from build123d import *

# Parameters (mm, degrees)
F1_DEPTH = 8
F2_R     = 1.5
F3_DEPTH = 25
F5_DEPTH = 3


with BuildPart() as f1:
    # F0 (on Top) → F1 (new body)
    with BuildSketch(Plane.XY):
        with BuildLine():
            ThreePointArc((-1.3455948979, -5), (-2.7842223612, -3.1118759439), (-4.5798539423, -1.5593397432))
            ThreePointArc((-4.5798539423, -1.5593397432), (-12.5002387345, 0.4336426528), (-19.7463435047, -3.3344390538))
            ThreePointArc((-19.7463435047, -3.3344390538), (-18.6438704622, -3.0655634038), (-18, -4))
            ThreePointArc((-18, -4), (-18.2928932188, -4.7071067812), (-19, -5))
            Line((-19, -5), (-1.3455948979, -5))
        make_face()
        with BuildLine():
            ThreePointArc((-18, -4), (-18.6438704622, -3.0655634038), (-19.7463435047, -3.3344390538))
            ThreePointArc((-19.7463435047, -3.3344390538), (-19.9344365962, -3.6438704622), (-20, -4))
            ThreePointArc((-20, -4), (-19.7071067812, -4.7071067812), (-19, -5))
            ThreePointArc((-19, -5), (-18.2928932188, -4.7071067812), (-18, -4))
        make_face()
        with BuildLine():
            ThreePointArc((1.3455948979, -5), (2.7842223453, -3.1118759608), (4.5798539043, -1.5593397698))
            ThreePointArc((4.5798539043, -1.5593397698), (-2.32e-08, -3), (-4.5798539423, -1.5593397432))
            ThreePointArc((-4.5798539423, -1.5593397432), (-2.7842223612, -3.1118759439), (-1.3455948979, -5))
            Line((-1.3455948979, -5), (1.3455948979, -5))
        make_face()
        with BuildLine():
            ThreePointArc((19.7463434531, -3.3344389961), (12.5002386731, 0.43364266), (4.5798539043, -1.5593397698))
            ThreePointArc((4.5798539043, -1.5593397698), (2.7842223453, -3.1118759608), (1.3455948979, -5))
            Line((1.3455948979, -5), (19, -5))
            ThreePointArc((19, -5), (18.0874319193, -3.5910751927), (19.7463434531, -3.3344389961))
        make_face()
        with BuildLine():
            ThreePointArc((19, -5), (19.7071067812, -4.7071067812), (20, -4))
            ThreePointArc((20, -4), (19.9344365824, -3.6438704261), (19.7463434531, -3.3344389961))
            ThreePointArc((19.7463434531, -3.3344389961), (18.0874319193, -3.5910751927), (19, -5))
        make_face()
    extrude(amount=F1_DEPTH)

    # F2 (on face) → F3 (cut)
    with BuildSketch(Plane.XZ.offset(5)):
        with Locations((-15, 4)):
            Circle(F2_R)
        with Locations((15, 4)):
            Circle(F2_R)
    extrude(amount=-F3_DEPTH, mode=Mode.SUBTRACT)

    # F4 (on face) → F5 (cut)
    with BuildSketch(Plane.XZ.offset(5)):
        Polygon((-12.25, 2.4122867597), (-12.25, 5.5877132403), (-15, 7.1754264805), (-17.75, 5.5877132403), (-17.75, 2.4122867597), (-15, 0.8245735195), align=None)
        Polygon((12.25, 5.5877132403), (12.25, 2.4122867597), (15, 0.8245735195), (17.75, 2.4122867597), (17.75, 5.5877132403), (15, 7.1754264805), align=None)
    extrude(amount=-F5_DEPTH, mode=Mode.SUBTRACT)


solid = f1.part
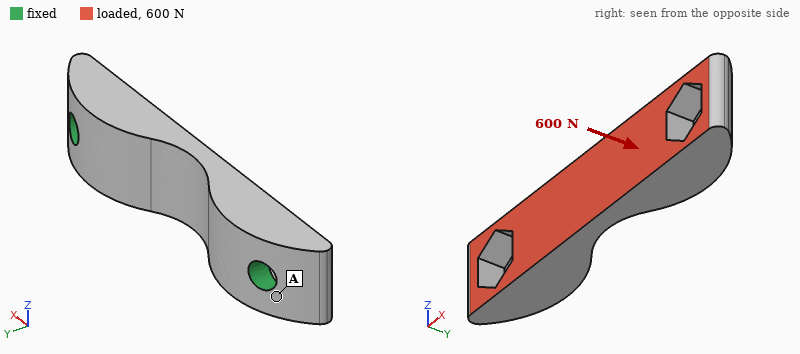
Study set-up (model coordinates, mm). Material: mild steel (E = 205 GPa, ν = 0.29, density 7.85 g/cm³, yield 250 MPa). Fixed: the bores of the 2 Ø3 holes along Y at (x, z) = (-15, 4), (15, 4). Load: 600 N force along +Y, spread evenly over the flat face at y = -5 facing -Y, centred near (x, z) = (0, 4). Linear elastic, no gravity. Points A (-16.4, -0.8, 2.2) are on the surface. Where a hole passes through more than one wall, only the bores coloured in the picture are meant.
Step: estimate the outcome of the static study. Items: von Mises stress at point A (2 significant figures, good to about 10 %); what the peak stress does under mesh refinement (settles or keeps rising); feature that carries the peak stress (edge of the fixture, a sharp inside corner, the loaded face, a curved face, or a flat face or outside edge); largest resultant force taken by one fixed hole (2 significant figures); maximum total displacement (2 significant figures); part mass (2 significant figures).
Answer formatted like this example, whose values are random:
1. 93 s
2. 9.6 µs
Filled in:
1. 16 MPa
2. keeps rising
3. edge of the fixture
4. 470 N
5. 5.4 µm
6. 8.7 g
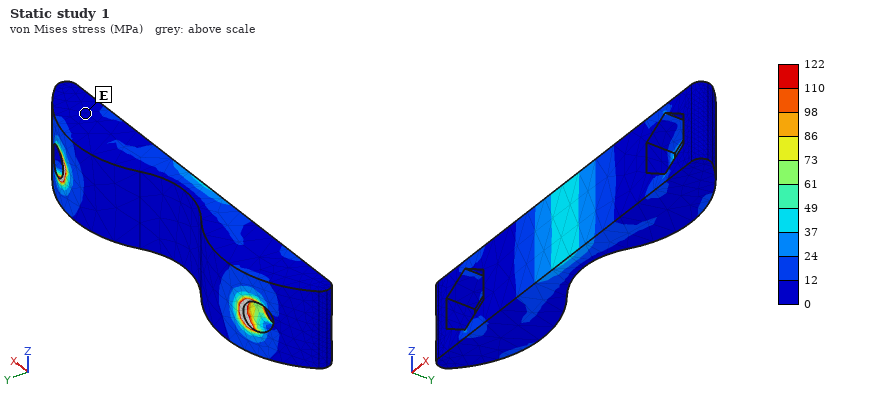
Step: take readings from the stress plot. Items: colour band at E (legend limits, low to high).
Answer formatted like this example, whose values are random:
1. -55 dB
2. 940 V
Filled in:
1. 0 to 12 MPa
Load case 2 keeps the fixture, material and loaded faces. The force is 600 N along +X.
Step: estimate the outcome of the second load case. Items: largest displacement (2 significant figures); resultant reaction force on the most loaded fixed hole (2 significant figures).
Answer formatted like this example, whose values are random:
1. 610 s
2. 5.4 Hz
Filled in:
1. 1.5 µm
2. 310 N
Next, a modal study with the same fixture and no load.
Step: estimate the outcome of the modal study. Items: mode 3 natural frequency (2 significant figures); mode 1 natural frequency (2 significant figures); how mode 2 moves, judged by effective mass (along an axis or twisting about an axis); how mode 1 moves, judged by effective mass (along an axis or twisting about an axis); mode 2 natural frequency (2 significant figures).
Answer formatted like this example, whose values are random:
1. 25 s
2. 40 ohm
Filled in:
1. 38 kHz
2. 22 kHz
3. along Y
4. along Z
5. 24 kHz
